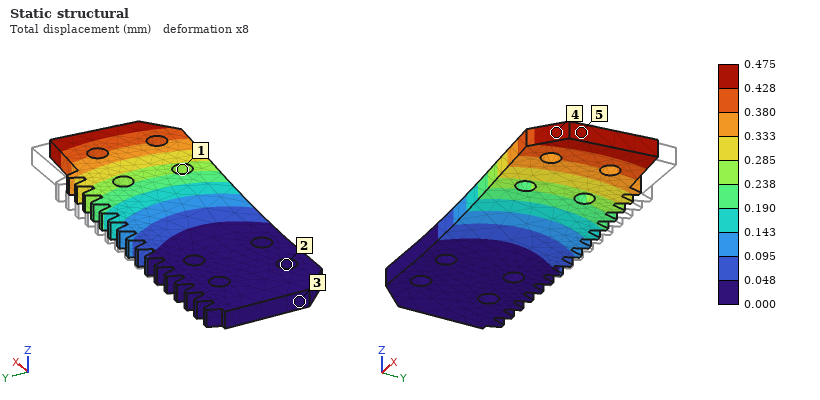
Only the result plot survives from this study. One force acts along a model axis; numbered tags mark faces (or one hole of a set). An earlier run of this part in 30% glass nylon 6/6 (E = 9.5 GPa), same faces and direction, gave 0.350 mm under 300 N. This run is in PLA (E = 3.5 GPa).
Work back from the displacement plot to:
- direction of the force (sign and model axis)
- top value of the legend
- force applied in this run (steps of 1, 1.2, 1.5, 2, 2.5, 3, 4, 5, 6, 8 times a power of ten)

-Y
0.475 mm
150 N
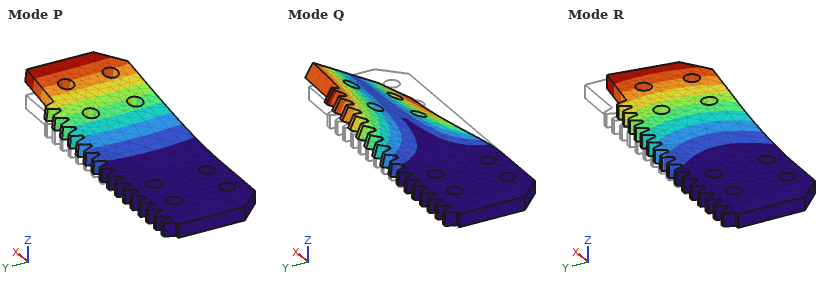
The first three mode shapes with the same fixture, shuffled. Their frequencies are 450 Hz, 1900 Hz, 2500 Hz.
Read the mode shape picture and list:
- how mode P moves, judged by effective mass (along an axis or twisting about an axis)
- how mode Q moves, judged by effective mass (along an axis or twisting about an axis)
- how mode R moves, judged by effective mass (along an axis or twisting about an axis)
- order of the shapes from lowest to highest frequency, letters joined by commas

along Z
twisting about X
along Y
P, Q, R
